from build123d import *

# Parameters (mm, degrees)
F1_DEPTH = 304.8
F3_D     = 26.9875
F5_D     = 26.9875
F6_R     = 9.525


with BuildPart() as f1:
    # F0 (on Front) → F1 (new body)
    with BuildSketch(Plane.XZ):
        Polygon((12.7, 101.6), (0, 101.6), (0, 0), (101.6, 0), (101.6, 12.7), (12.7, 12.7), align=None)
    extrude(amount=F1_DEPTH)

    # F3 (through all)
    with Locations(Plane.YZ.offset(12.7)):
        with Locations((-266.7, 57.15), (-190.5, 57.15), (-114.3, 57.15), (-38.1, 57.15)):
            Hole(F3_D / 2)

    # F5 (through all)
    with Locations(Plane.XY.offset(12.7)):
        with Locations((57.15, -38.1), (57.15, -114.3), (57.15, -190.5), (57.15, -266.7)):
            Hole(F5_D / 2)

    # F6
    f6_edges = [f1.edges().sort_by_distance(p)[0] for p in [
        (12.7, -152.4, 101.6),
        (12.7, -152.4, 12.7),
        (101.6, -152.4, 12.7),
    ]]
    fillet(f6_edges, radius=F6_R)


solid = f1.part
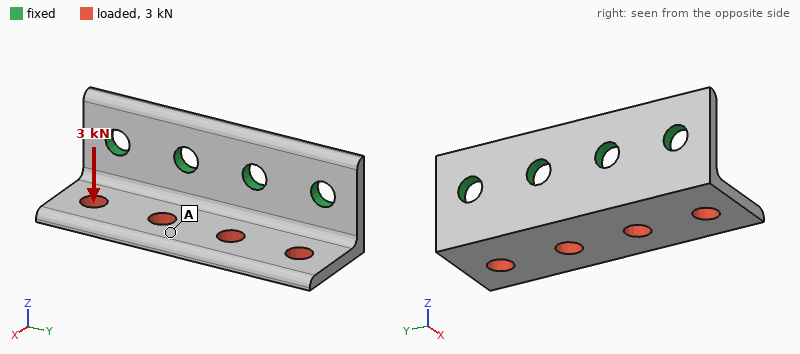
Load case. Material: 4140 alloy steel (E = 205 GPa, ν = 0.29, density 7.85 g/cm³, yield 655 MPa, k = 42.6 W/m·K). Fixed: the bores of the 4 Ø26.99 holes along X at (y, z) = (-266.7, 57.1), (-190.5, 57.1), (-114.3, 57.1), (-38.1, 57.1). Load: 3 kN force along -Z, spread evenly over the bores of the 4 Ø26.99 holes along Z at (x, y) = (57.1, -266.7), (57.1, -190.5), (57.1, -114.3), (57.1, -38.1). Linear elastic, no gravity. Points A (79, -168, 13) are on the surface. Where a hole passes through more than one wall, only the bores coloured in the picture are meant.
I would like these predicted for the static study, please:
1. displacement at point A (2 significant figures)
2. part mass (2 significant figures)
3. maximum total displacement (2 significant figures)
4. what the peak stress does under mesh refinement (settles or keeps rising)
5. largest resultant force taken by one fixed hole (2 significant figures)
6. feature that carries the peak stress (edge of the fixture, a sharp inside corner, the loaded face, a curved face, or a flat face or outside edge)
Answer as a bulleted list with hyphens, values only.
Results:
- 51 µm
- 5.3 kg
- 70 µm
- keeps rising
- 790 N
- edge of the fixture
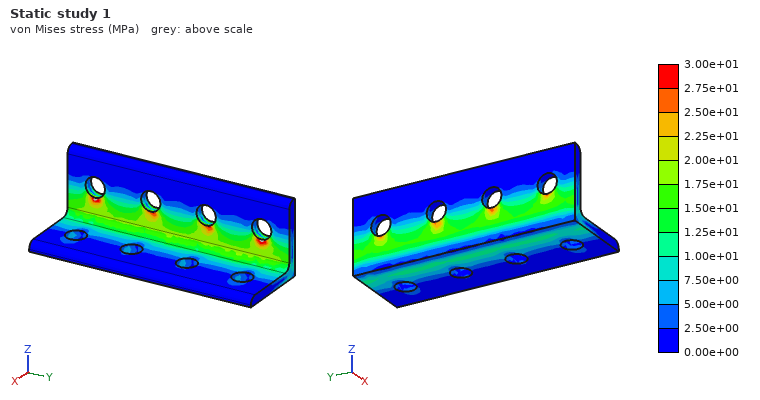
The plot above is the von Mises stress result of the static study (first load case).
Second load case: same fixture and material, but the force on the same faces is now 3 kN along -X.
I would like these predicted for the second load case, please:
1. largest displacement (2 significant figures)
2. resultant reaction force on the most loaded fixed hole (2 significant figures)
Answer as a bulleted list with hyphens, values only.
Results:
- 25 µm
- 750 N
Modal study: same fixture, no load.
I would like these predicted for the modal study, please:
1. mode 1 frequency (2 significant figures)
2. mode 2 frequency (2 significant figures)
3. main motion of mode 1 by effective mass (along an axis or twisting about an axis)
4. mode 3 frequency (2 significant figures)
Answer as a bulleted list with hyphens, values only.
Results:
- 770 Hz
- 1000 Hz
- along Z
- 2000 Hz
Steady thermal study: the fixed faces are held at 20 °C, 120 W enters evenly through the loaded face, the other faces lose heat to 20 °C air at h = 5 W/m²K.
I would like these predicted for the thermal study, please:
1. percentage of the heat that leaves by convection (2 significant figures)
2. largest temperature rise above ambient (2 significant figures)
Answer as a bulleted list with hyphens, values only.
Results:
- 14 %
- 67 K
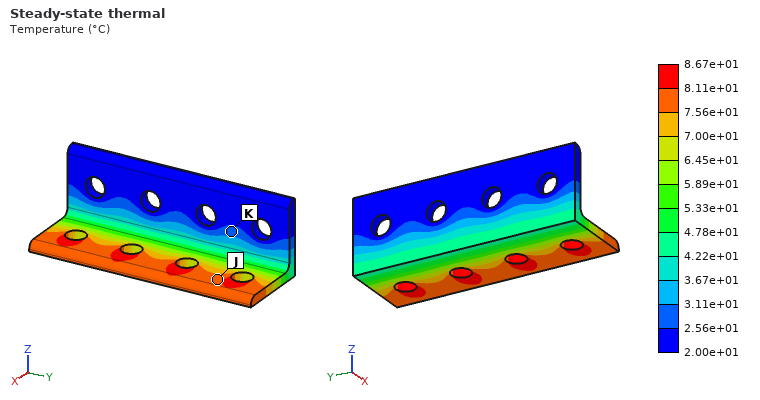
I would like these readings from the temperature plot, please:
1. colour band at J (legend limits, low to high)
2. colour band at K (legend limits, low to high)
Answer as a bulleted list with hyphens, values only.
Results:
- 7.56e+01 to 8.11e+01 °C
- 2.56e+01 to 3.11e+01 °C
